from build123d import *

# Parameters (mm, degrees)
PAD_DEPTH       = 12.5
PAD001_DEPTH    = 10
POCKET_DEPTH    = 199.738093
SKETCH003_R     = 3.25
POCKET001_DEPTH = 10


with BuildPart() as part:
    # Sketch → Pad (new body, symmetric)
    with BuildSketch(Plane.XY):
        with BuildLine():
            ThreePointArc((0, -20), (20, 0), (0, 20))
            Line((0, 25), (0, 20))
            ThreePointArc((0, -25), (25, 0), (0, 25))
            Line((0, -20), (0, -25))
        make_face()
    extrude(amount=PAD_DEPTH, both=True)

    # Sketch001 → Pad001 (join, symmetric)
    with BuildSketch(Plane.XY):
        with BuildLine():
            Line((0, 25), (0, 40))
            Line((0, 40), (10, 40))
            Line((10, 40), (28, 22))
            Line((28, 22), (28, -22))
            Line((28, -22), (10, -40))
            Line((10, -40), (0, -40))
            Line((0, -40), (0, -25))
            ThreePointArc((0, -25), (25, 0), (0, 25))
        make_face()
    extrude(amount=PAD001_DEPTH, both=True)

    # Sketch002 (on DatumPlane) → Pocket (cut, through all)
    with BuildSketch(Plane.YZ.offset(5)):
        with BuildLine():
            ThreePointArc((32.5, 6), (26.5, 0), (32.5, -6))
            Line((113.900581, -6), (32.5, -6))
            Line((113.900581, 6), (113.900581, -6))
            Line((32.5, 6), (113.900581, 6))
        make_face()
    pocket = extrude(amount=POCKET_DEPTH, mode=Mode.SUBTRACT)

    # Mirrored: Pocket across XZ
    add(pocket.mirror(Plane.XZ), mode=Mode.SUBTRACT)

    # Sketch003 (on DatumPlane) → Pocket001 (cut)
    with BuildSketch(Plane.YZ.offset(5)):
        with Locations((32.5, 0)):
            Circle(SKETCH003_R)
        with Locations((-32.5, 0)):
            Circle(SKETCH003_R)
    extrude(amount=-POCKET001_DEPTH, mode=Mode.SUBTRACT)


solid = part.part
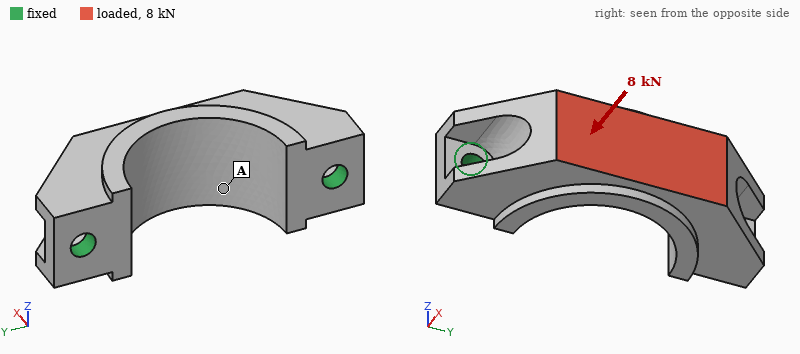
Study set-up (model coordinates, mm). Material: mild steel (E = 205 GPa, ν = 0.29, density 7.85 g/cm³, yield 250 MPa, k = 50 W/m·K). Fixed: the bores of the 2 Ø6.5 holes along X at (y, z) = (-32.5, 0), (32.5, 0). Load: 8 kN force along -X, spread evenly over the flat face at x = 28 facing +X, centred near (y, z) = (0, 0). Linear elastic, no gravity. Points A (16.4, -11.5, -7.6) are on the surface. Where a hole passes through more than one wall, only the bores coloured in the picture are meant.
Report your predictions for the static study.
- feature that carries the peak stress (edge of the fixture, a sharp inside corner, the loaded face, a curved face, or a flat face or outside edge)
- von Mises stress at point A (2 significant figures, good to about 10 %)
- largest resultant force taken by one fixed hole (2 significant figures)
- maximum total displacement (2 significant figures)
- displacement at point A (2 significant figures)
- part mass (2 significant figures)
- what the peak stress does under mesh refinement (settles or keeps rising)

edge of the fixture
27 MPa
5.2 kN
10 µm
7.8 µm
190 g
keeps rising
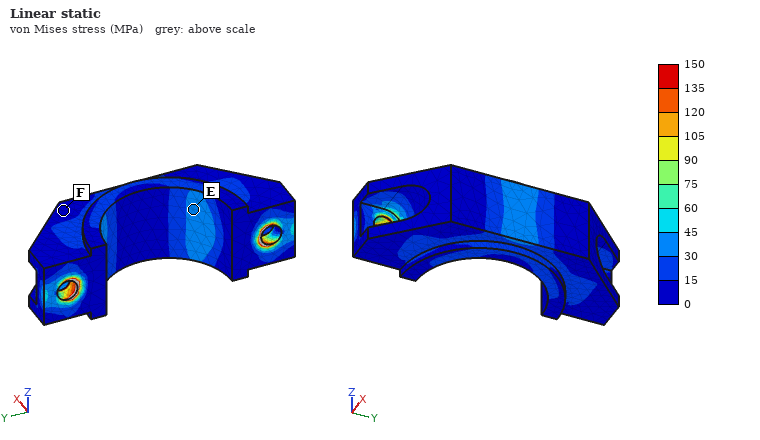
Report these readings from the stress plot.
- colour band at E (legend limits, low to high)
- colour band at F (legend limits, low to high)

30 to 45 MPa
0 to 15 MPa
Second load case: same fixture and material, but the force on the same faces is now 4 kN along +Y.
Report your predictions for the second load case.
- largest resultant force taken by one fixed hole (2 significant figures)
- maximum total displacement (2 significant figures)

2.5 kN
6.5 µm
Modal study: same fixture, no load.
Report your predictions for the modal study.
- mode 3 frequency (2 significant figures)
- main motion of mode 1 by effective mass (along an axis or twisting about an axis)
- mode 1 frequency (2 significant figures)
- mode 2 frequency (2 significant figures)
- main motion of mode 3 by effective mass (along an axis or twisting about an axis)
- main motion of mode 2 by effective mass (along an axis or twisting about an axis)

12 kHz
along Z
4600 Hz
11 kHz
along Y
twisting about X
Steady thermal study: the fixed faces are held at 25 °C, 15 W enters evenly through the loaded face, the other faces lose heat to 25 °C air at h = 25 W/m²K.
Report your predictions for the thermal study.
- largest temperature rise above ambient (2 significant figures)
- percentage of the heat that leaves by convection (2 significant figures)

20 K
12 %
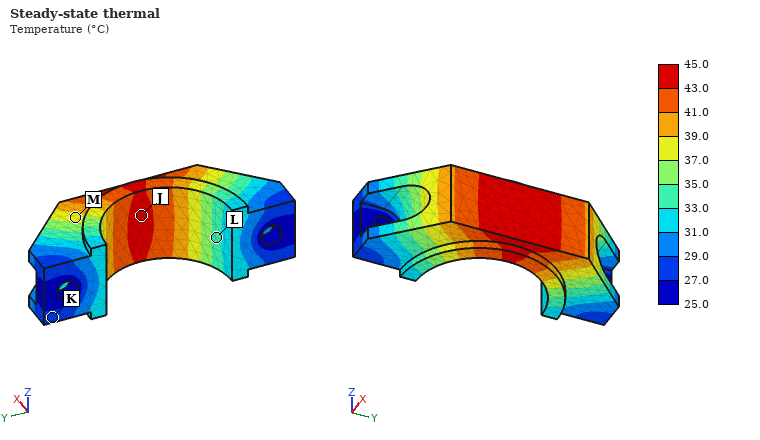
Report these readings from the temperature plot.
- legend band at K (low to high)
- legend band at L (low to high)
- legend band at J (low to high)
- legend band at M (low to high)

27.0 to 29.0 °C
33.0 to 35.0 °C
43.0 to 45.0 °C
37.0 to 39.0 °C
